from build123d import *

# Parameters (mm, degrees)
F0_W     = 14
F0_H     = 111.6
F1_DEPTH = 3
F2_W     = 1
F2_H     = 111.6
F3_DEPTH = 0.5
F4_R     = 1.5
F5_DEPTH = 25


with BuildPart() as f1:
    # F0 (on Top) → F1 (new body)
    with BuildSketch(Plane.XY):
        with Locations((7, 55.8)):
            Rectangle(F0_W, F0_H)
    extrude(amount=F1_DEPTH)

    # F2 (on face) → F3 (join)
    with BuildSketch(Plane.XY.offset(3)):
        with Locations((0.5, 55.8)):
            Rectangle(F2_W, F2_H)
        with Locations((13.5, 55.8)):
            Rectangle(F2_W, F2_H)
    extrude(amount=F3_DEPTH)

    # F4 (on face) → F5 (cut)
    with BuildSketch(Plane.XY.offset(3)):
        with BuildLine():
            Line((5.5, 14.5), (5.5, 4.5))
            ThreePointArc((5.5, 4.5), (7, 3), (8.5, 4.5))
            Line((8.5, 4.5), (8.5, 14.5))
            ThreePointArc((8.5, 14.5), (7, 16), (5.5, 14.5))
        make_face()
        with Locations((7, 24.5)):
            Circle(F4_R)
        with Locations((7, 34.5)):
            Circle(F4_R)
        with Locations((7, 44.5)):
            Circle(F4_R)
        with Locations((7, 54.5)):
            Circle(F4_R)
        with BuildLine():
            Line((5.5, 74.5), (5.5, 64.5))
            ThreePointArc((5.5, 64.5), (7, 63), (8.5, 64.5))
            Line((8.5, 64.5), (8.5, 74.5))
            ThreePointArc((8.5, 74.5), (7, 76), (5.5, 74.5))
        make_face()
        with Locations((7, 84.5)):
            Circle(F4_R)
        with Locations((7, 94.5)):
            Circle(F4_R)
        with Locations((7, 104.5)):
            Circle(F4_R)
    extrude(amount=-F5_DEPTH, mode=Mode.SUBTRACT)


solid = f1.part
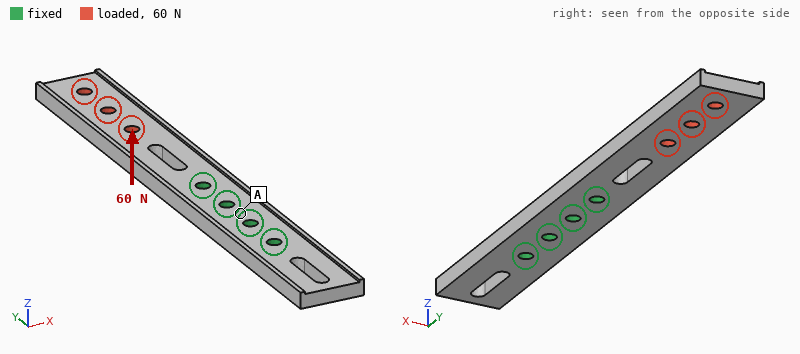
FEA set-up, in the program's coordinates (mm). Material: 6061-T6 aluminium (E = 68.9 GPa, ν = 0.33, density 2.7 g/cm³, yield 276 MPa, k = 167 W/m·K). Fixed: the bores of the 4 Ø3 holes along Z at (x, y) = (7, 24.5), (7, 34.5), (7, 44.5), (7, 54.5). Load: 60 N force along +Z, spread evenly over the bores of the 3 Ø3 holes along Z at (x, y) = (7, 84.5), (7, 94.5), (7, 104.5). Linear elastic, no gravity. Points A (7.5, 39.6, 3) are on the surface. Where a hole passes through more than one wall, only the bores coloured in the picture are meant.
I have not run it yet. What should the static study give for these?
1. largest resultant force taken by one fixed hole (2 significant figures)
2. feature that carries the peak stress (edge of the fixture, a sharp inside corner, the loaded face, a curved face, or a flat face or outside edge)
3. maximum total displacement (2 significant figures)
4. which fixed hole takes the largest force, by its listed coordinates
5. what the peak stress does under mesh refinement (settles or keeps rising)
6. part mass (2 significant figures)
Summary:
130 N
edge of the fixture
0.99 mm
(7, 54.5)
keeps rising
12 g
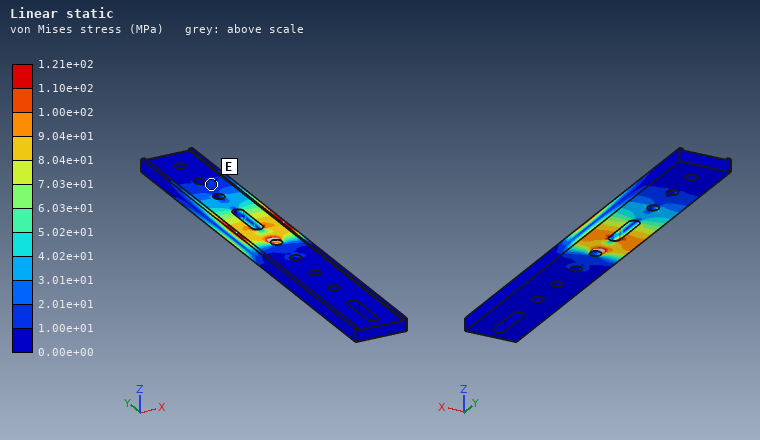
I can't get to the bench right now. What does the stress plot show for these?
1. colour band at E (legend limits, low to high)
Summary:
1.00e+01 to 2.01e+01 MPa
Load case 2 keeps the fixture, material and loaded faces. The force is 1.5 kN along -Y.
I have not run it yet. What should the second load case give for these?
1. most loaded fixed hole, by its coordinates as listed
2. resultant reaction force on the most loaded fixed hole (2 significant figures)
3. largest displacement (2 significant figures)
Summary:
(7, 54.5)
1.2 kN
52 µm
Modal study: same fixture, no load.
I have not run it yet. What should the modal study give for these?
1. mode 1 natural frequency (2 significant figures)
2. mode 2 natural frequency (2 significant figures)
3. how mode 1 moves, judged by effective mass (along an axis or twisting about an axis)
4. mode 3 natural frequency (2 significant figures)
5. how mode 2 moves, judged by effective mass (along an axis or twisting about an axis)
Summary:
760 Hz
2900 Hz
along Z
4400 Hz
along X
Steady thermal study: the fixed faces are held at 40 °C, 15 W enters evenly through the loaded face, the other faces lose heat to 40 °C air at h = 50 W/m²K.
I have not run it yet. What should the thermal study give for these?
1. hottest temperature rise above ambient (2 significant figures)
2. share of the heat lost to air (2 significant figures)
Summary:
71 K
31 %
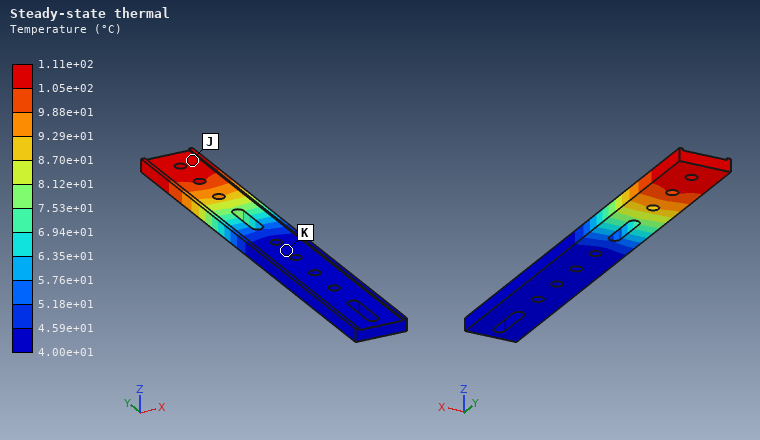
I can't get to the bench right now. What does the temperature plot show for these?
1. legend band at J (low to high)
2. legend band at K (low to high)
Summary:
1.05e+02 to 1.11e+02 °C
4.00e+01 to 4.59e+01 °C
